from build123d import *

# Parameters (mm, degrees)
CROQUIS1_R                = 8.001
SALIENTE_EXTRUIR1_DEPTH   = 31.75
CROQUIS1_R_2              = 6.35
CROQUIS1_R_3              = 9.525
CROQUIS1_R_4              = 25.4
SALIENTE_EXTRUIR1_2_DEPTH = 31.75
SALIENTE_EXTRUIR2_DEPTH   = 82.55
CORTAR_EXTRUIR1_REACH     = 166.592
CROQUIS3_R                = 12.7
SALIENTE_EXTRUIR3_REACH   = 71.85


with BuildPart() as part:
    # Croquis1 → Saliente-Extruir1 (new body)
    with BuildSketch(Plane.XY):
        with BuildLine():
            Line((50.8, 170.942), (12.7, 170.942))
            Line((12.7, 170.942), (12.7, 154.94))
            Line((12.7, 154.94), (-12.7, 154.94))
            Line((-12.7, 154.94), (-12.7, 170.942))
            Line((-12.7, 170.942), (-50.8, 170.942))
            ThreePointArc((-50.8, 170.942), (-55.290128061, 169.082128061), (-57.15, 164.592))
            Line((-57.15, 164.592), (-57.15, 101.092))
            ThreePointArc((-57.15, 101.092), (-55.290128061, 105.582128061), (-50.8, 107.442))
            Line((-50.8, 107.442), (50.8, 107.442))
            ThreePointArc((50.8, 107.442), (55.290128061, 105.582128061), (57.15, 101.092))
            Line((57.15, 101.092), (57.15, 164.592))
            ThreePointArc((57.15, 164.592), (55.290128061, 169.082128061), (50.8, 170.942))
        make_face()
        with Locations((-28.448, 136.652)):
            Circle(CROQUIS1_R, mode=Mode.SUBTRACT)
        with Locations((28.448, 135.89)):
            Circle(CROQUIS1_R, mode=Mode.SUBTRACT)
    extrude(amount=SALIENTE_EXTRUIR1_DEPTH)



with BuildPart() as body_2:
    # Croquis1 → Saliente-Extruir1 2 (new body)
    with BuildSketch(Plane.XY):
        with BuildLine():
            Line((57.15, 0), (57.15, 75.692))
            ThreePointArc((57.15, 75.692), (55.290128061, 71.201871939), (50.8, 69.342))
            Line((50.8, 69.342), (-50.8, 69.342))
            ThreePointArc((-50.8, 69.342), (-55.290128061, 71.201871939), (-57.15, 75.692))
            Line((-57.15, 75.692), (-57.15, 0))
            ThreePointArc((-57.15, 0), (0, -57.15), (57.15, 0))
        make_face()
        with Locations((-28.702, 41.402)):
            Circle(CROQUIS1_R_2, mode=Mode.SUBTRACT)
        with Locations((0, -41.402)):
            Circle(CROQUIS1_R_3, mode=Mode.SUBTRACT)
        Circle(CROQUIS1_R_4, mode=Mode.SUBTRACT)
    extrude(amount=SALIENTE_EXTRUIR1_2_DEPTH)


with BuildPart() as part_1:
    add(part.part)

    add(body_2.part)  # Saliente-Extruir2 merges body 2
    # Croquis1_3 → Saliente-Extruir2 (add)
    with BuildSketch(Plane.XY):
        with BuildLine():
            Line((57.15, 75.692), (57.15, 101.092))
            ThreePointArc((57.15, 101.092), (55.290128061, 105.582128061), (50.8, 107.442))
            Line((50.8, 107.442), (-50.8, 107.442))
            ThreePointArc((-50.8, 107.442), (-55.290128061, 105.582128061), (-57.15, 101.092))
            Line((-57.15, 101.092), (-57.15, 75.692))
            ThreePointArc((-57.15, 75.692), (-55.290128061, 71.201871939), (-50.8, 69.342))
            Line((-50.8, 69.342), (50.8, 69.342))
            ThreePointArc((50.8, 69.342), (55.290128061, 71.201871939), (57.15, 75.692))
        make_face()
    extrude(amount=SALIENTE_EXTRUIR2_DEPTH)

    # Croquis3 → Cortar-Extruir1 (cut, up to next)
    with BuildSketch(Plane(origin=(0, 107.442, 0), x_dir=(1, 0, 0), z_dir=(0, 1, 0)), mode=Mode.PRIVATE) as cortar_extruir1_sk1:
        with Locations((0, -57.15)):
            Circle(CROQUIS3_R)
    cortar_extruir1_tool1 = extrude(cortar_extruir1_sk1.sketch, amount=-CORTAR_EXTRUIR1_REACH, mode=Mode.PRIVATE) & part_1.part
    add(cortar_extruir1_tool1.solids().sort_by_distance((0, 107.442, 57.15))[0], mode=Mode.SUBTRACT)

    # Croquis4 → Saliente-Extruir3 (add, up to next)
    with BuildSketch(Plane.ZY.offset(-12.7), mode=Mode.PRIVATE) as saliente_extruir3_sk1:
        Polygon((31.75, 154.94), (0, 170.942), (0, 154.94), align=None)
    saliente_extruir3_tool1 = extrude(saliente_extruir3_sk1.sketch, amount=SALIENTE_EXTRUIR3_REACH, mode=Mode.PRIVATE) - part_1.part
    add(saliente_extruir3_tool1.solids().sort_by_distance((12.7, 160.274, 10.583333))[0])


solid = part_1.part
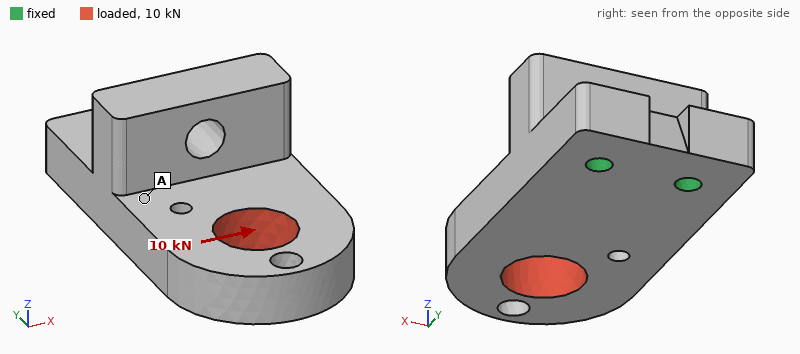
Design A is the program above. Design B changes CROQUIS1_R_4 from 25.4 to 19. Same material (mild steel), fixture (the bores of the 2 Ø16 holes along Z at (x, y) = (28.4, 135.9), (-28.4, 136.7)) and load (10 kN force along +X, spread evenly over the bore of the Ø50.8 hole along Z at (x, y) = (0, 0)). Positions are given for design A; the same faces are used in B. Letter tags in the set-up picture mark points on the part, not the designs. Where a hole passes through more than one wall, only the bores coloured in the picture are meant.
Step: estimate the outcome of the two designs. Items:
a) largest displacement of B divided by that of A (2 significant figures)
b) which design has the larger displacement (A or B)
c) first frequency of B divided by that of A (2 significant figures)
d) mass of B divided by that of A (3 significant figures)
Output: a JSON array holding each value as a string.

["0.92", "A", "0.96", "1.03"]
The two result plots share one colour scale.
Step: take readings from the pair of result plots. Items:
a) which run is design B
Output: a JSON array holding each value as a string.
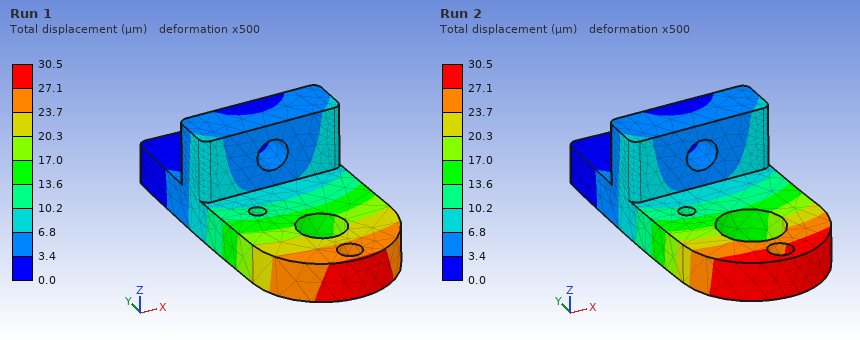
["Run 1"]
